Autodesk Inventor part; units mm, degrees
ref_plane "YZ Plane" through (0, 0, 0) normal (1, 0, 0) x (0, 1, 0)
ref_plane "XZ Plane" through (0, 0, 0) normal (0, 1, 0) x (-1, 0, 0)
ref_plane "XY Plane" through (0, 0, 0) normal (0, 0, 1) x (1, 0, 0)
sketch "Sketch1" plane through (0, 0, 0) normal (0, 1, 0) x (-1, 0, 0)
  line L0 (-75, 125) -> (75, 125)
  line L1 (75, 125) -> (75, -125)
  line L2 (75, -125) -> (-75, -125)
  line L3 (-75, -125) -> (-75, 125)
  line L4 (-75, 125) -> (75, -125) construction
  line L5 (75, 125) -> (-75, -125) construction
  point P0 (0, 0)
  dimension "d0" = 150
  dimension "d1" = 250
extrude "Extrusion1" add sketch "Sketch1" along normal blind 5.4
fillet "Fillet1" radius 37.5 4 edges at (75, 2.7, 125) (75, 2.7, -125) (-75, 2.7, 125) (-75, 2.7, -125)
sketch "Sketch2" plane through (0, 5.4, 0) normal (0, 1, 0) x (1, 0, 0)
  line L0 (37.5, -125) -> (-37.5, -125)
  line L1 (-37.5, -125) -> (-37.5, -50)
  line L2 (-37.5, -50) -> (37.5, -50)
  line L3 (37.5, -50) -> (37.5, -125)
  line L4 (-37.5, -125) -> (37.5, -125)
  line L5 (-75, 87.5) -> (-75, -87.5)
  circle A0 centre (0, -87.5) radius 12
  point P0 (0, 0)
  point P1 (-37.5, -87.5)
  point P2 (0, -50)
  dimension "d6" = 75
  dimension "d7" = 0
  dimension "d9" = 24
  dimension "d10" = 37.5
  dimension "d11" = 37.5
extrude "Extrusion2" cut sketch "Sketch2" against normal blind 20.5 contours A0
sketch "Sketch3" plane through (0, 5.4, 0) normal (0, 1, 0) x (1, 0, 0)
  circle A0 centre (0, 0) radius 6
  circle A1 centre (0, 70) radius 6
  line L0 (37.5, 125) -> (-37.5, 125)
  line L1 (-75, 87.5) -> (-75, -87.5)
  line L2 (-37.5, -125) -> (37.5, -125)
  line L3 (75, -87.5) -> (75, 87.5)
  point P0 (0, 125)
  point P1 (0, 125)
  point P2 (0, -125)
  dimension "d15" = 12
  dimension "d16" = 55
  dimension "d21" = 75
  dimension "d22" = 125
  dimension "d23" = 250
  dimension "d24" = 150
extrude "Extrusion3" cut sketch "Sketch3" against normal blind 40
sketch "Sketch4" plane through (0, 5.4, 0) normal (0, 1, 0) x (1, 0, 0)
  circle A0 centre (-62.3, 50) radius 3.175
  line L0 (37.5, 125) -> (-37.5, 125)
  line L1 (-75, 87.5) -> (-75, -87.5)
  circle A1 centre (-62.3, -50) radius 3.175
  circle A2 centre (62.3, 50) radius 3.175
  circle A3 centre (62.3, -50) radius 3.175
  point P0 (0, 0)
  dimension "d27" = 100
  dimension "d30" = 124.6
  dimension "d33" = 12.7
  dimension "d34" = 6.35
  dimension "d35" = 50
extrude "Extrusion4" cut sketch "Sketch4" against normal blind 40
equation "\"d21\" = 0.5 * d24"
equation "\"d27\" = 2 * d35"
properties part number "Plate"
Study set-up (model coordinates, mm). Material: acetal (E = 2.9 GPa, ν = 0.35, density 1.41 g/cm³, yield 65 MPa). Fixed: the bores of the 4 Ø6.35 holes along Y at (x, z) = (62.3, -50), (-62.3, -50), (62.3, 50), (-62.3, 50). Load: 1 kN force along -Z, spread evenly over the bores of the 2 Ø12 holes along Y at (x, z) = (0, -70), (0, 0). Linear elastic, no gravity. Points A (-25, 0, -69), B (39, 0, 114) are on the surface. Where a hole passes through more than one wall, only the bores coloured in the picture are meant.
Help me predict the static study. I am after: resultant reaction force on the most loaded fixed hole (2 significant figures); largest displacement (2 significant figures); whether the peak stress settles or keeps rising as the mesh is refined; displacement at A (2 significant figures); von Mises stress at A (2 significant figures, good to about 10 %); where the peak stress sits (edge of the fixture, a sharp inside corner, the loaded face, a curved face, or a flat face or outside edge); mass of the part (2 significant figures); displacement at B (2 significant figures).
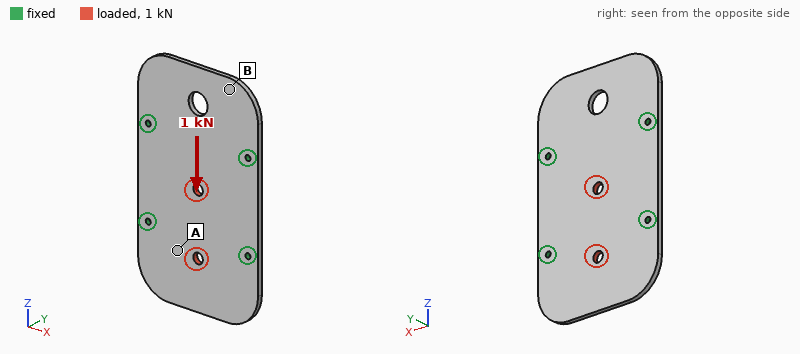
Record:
280 N
48 µm
keeps rising
29 µm
0.83 MPa
edge of the fixture
270 g
12 µm
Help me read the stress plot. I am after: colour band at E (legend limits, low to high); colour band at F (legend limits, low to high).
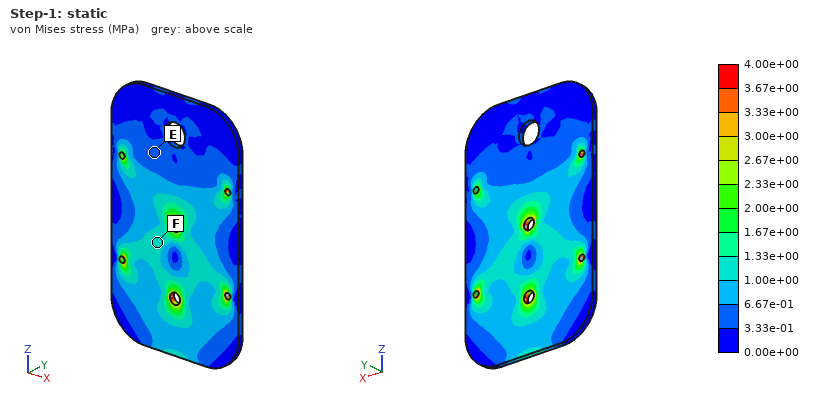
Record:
3.33e-01 to 6.67e-01 MPa
1.00e+00 to 1.33e+00 MPa
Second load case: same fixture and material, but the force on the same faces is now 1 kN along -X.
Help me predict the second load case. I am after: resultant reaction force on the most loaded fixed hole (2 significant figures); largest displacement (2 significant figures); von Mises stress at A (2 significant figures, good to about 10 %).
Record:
350 N
43 µm
1.4 MPa
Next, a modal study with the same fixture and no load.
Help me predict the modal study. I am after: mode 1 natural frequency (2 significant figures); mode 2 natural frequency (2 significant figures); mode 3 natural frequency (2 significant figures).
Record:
190 Hz
190 Hz
390 Hz
